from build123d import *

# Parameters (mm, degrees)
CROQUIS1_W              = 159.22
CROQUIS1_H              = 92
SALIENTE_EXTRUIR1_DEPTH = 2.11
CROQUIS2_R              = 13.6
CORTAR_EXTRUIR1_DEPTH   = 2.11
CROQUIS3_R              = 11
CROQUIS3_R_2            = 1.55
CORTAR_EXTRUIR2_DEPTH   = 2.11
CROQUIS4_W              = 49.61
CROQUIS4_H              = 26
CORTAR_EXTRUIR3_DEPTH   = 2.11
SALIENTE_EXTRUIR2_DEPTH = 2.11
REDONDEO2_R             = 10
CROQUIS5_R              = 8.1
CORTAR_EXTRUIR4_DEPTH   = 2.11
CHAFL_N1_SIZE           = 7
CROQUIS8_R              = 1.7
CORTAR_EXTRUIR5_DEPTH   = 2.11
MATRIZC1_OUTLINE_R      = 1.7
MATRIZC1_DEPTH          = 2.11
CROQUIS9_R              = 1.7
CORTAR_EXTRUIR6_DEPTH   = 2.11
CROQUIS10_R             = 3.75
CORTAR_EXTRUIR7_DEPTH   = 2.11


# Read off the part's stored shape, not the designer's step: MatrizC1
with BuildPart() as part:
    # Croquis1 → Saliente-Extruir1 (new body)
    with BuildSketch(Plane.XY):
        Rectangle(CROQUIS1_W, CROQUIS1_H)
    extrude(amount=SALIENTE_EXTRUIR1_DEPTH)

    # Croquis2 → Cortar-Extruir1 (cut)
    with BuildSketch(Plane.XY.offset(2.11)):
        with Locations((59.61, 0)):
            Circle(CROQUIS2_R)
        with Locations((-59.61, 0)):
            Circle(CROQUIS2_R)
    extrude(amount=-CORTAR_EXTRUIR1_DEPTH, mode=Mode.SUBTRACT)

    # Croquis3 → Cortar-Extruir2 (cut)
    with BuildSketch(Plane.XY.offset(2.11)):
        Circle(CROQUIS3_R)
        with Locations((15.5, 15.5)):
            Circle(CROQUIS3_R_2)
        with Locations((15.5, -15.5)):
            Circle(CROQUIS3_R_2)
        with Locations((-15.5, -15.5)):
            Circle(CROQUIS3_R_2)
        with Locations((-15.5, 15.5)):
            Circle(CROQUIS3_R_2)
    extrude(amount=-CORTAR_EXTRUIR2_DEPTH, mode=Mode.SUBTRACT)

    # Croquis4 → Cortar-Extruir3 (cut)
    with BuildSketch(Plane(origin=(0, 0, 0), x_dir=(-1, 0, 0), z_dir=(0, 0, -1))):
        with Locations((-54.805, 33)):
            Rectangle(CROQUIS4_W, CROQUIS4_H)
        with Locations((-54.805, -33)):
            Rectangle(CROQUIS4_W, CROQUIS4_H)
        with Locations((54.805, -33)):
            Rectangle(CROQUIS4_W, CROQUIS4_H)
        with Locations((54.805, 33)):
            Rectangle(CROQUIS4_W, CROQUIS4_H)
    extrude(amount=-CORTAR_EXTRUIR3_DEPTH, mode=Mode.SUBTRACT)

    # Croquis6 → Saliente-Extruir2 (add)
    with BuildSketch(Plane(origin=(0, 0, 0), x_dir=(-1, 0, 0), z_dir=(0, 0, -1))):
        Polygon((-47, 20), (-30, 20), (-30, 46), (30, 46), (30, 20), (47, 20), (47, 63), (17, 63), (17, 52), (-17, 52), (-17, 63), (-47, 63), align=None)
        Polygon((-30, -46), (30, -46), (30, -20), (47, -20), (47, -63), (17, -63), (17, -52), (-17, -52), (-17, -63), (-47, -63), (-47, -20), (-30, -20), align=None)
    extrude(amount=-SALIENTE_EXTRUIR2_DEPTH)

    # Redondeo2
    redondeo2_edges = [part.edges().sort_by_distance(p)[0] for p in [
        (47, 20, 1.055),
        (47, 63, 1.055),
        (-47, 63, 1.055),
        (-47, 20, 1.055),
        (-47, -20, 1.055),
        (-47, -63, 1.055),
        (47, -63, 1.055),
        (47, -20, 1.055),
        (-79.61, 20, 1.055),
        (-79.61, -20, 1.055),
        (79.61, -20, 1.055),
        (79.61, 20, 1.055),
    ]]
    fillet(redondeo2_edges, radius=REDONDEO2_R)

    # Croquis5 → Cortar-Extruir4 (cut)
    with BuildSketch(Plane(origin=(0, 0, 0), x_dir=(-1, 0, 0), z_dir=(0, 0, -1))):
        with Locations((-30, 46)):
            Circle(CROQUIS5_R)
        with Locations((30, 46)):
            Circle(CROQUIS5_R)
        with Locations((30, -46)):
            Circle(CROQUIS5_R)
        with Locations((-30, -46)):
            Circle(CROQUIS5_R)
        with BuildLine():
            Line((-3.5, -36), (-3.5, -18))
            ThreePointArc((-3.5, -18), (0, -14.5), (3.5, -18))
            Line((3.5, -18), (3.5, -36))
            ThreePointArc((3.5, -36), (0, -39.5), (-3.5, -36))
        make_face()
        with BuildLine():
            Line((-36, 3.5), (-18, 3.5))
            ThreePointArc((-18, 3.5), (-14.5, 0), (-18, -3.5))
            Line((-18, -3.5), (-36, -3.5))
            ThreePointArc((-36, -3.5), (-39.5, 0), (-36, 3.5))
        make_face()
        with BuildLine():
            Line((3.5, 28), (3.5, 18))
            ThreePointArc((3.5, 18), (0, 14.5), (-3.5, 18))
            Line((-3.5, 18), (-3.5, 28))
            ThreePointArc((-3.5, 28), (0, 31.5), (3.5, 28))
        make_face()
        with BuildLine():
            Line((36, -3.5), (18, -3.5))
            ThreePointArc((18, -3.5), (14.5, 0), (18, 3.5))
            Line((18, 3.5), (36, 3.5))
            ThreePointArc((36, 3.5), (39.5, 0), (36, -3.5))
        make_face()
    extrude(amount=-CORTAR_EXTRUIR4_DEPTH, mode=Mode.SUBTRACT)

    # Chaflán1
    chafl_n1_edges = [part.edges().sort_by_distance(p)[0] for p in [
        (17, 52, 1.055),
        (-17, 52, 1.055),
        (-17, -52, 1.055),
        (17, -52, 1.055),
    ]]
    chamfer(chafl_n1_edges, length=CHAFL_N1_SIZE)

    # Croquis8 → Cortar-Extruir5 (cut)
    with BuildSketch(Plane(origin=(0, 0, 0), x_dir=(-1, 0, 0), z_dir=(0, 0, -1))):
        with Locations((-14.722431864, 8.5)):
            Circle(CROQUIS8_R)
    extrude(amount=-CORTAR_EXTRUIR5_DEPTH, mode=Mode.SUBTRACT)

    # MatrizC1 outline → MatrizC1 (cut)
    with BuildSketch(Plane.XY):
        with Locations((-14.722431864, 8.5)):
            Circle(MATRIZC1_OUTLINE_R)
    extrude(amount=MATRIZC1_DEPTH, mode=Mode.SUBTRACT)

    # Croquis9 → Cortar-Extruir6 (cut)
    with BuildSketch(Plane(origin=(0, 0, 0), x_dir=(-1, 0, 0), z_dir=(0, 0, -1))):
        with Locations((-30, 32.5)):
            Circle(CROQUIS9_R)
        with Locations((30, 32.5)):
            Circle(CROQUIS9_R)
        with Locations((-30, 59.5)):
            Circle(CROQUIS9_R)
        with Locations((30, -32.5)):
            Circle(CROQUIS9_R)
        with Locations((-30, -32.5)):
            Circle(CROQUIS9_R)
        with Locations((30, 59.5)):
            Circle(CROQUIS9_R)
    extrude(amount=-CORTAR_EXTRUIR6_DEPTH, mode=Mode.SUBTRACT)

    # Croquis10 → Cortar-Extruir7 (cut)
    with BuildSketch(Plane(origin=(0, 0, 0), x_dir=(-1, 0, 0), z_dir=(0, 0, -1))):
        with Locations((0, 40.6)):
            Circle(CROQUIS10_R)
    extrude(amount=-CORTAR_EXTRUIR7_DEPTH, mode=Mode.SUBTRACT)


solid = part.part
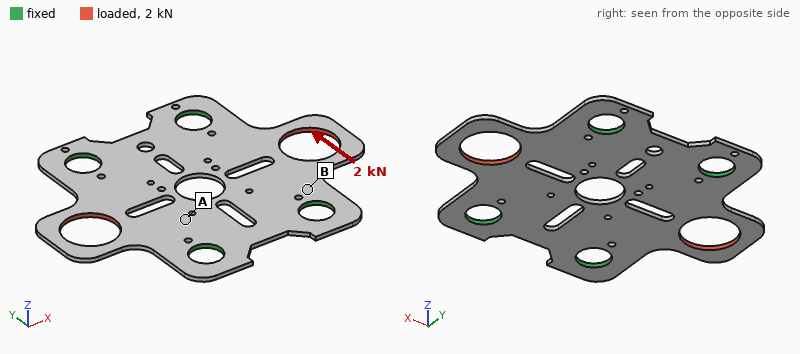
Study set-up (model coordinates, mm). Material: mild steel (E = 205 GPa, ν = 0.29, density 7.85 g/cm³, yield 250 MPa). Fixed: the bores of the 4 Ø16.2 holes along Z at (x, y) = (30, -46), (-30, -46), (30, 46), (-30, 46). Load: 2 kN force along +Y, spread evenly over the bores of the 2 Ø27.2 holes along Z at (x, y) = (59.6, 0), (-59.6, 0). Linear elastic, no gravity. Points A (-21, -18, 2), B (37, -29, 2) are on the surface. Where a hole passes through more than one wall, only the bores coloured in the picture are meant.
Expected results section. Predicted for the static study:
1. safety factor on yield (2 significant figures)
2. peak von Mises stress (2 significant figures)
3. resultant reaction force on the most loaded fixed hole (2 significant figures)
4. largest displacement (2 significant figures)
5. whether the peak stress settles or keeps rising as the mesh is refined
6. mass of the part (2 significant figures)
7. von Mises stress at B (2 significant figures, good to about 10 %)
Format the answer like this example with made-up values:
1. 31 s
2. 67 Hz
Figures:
1. 2.4
2. 100 MPa
3. 580 N
4. 24 µm
5. settles
6. 180 g
7. 16 MPa
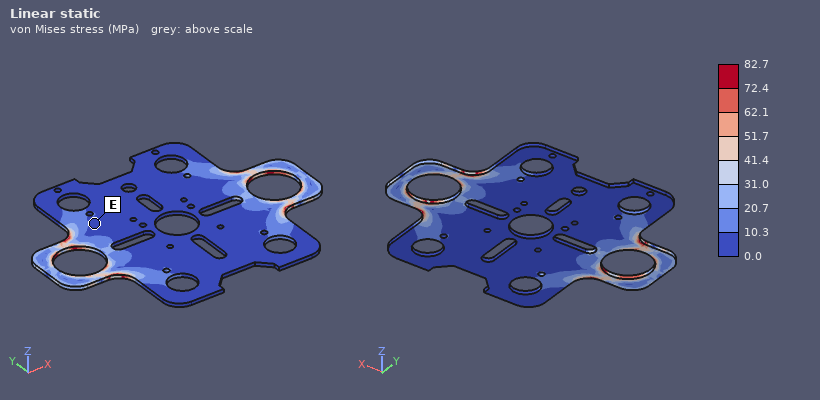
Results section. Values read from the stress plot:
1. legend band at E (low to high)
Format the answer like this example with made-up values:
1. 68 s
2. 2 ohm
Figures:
1. 0.0 to 10.3 MPa
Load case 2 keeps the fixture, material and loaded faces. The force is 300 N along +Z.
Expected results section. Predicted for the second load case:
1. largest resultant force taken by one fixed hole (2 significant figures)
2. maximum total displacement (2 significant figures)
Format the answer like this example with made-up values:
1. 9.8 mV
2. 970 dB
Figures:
1. 75 N
2. 0.57 mm
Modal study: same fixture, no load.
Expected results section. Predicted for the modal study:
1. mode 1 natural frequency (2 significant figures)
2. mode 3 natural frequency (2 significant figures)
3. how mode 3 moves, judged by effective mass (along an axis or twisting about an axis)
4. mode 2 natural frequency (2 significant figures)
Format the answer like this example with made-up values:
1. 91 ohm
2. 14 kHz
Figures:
1. 770 Hz
2. 1600 Hz
3. along Z
4. 780 Hz
